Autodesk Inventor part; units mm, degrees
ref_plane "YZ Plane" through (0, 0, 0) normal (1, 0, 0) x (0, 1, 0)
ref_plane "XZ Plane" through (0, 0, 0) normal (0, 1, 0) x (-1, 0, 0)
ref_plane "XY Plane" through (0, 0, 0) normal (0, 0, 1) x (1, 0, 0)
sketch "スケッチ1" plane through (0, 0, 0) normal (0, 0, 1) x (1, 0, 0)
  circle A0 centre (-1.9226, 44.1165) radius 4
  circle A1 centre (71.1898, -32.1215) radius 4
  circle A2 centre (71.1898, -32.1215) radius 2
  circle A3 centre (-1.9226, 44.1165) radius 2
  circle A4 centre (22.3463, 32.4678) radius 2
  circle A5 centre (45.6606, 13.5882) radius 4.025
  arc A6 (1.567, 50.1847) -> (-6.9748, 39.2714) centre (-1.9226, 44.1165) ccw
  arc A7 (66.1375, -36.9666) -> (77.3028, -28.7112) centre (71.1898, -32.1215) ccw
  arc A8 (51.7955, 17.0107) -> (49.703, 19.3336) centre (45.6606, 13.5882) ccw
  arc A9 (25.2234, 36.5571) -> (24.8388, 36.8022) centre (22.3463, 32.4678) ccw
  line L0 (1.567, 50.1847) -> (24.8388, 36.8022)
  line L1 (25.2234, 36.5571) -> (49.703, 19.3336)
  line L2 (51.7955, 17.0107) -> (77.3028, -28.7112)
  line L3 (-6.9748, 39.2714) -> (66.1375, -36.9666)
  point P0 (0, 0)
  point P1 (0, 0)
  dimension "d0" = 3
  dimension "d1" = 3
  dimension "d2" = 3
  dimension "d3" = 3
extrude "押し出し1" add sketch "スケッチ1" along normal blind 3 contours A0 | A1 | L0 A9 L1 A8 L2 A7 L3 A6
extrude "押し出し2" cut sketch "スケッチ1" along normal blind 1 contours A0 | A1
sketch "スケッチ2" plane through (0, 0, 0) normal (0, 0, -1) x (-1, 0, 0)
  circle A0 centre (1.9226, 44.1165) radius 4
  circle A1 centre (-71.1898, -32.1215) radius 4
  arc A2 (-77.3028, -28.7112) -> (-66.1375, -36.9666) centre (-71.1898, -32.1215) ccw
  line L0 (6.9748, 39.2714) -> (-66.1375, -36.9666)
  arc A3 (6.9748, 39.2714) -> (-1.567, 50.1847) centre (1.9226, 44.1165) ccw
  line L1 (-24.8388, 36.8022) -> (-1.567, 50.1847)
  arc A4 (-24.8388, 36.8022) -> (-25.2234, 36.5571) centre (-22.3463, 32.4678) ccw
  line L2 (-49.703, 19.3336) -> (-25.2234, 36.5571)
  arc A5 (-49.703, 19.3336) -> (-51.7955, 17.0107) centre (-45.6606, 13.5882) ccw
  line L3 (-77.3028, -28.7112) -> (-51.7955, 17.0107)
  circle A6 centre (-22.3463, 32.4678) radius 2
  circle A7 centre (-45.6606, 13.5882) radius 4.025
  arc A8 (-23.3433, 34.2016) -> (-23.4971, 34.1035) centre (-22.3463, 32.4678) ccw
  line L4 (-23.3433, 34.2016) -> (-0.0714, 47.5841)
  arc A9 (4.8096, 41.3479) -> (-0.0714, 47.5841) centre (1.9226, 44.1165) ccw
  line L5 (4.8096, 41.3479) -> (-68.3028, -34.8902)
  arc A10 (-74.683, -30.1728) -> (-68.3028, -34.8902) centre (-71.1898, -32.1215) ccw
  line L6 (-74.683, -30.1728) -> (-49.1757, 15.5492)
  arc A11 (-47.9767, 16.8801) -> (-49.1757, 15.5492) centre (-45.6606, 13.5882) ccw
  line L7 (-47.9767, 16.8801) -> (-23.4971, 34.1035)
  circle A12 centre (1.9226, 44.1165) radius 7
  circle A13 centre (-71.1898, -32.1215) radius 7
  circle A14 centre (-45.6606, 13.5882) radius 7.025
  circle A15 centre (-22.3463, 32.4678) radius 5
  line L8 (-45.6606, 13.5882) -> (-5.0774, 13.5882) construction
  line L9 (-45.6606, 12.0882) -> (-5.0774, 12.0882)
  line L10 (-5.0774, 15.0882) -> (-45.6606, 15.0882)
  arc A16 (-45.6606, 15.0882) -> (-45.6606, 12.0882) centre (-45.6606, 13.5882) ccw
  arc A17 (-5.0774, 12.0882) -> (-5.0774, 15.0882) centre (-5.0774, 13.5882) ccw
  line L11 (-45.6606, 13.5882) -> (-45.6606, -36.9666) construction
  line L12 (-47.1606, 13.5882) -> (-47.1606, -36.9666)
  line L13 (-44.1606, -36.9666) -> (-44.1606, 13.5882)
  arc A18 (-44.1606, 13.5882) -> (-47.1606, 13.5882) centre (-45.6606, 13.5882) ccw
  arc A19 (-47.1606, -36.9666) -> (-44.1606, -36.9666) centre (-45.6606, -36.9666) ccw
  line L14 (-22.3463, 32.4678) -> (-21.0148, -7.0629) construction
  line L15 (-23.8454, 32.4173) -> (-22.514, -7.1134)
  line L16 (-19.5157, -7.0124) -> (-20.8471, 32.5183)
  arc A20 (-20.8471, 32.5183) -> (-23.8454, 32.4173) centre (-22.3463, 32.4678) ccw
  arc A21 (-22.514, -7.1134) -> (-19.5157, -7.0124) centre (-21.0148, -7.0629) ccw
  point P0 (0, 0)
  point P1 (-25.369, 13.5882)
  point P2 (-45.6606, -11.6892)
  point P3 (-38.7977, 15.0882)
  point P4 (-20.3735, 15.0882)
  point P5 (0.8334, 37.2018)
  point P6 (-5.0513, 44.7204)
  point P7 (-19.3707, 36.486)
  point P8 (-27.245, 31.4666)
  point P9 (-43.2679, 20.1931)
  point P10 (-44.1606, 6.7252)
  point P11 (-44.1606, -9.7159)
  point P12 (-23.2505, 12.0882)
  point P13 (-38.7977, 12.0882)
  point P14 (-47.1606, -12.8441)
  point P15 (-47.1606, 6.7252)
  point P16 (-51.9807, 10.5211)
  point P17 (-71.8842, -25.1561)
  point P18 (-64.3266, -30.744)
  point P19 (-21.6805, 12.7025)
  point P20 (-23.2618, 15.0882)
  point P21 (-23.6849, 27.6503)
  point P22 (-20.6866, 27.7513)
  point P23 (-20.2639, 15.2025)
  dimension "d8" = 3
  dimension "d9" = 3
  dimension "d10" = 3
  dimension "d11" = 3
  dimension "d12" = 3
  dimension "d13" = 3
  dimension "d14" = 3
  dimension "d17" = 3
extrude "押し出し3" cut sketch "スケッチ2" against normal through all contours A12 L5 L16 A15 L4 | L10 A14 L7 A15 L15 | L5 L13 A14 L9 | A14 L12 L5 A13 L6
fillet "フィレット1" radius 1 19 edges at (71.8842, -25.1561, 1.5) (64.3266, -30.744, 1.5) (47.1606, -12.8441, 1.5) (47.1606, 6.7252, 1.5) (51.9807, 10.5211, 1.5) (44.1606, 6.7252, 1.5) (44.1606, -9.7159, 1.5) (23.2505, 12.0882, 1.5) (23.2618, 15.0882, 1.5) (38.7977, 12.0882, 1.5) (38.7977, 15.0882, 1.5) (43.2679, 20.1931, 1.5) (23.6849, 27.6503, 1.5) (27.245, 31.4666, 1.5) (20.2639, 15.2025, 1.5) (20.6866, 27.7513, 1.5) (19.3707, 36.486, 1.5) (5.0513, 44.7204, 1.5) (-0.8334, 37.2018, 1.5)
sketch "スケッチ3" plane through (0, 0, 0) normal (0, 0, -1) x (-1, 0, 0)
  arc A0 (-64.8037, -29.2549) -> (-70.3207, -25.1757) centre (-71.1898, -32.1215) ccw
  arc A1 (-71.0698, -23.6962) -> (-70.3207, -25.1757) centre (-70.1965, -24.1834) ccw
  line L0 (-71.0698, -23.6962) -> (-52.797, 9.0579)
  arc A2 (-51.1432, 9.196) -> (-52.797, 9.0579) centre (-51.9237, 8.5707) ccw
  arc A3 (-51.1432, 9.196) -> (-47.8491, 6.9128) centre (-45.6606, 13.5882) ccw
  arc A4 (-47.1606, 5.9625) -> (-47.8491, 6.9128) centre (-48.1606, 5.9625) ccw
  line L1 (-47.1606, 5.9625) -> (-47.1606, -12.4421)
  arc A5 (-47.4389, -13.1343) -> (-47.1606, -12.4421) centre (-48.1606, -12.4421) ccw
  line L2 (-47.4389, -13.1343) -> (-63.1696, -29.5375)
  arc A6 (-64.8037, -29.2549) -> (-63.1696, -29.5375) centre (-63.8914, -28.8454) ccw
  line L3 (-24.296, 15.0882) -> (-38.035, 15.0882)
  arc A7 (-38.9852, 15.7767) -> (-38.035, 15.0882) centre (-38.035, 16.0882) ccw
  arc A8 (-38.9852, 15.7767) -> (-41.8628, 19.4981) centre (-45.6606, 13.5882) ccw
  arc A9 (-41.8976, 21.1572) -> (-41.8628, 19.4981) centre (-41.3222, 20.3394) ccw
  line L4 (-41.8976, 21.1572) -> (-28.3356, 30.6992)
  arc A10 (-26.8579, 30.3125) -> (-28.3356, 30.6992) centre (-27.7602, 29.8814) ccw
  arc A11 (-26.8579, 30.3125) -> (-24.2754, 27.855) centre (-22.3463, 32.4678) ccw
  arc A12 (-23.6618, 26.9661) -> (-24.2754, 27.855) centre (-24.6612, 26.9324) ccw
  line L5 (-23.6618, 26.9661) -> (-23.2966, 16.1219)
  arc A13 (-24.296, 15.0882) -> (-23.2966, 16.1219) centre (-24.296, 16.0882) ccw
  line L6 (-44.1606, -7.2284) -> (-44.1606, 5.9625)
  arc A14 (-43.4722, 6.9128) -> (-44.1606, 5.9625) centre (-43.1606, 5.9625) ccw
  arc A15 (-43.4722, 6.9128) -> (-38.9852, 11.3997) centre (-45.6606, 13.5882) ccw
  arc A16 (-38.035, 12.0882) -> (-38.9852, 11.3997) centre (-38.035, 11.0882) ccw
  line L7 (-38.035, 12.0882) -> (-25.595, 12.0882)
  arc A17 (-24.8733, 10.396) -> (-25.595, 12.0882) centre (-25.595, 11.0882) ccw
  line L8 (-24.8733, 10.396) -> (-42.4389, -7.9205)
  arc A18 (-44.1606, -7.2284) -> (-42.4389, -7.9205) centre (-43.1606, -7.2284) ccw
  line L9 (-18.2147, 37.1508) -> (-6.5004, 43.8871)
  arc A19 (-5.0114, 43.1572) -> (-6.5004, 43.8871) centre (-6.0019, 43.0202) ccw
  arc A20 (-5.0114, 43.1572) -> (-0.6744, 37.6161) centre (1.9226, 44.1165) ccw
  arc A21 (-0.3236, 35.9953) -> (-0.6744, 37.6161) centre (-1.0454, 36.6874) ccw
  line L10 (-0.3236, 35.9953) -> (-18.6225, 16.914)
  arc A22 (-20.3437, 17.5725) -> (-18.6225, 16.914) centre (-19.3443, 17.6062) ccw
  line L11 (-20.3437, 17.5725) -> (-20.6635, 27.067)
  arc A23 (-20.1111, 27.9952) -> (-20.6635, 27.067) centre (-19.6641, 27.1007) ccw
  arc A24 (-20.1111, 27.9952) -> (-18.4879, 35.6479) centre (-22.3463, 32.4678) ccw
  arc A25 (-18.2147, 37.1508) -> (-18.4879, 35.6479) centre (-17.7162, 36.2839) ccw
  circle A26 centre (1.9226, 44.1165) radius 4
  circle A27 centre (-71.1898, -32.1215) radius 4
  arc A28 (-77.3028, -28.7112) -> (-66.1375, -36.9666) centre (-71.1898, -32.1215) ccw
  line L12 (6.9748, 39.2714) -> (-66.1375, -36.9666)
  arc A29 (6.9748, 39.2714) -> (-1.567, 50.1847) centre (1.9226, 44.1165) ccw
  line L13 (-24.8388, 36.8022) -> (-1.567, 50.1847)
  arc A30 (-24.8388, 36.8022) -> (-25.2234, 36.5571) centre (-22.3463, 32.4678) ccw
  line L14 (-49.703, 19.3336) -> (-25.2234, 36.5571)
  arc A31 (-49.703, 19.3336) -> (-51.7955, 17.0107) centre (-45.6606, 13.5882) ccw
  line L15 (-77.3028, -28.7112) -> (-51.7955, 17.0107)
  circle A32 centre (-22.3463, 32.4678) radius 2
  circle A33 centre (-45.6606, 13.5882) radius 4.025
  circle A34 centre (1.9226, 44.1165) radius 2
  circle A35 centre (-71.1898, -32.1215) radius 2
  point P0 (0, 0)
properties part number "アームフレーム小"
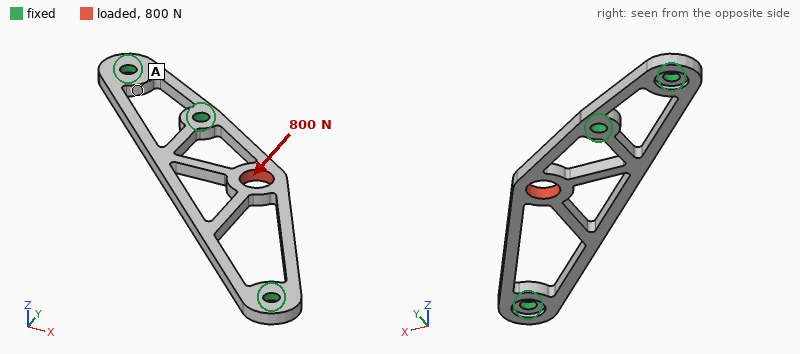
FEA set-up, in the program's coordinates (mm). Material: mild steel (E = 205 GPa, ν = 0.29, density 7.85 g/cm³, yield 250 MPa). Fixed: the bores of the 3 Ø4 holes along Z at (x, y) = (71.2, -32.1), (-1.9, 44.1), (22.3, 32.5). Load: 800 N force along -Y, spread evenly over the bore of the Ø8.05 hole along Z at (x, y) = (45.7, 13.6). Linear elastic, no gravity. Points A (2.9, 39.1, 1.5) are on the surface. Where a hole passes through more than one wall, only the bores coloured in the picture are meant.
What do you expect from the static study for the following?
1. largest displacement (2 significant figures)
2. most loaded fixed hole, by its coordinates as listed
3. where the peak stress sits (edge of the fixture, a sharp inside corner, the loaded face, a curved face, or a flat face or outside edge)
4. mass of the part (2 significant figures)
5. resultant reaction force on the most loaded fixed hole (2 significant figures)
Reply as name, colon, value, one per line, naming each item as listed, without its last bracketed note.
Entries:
largest displacement: 49 µm
most loaded fixed hole, by its coordinates as listed: (22.3, 32.5)
where the peak stress sits: a curved face
mass of the part: 27 g
resultant reaction force on the most loaded fixed hole: 560 N
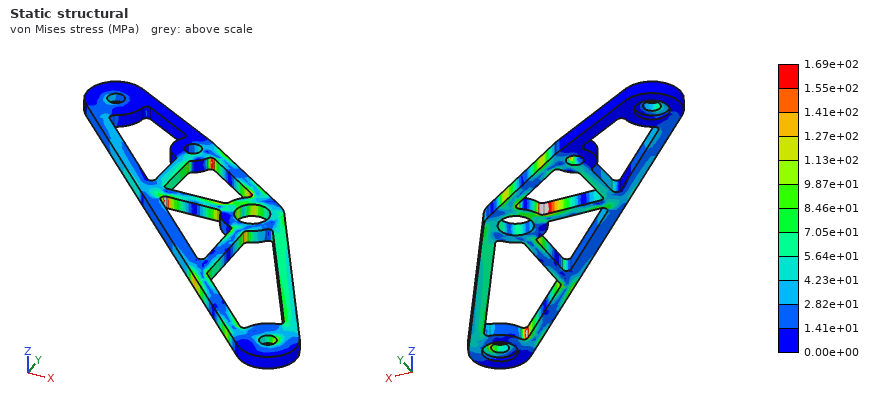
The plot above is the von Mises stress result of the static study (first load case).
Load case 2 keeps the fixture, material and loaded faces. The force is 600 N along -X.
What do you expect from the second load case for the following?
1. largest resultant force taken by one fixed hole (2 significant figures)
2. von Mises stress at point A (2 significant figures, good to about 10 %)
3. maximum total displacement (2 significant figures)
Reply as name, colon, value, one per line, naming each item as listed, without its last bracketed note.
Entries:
largest resultant force taken by one fixed hole: 360 N
von Mises stress at point A: 13 MPa
maximum total displacement: 28 µm
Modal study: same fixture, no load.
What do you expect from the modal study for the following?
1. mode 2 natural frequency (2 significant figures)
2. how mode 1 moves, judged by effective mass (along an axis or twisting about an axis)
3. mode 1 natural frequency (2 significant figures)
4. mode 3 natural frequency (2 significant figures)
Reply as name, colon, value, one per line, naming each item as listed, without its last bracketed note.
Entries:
mode 2 natural frequency: 2800 Hz
how mode 1 moves, judged by effective mass: along Z
mode 1 natural frequency: 2100 Hz
mode 3 natural frequency: 5300 Hz
